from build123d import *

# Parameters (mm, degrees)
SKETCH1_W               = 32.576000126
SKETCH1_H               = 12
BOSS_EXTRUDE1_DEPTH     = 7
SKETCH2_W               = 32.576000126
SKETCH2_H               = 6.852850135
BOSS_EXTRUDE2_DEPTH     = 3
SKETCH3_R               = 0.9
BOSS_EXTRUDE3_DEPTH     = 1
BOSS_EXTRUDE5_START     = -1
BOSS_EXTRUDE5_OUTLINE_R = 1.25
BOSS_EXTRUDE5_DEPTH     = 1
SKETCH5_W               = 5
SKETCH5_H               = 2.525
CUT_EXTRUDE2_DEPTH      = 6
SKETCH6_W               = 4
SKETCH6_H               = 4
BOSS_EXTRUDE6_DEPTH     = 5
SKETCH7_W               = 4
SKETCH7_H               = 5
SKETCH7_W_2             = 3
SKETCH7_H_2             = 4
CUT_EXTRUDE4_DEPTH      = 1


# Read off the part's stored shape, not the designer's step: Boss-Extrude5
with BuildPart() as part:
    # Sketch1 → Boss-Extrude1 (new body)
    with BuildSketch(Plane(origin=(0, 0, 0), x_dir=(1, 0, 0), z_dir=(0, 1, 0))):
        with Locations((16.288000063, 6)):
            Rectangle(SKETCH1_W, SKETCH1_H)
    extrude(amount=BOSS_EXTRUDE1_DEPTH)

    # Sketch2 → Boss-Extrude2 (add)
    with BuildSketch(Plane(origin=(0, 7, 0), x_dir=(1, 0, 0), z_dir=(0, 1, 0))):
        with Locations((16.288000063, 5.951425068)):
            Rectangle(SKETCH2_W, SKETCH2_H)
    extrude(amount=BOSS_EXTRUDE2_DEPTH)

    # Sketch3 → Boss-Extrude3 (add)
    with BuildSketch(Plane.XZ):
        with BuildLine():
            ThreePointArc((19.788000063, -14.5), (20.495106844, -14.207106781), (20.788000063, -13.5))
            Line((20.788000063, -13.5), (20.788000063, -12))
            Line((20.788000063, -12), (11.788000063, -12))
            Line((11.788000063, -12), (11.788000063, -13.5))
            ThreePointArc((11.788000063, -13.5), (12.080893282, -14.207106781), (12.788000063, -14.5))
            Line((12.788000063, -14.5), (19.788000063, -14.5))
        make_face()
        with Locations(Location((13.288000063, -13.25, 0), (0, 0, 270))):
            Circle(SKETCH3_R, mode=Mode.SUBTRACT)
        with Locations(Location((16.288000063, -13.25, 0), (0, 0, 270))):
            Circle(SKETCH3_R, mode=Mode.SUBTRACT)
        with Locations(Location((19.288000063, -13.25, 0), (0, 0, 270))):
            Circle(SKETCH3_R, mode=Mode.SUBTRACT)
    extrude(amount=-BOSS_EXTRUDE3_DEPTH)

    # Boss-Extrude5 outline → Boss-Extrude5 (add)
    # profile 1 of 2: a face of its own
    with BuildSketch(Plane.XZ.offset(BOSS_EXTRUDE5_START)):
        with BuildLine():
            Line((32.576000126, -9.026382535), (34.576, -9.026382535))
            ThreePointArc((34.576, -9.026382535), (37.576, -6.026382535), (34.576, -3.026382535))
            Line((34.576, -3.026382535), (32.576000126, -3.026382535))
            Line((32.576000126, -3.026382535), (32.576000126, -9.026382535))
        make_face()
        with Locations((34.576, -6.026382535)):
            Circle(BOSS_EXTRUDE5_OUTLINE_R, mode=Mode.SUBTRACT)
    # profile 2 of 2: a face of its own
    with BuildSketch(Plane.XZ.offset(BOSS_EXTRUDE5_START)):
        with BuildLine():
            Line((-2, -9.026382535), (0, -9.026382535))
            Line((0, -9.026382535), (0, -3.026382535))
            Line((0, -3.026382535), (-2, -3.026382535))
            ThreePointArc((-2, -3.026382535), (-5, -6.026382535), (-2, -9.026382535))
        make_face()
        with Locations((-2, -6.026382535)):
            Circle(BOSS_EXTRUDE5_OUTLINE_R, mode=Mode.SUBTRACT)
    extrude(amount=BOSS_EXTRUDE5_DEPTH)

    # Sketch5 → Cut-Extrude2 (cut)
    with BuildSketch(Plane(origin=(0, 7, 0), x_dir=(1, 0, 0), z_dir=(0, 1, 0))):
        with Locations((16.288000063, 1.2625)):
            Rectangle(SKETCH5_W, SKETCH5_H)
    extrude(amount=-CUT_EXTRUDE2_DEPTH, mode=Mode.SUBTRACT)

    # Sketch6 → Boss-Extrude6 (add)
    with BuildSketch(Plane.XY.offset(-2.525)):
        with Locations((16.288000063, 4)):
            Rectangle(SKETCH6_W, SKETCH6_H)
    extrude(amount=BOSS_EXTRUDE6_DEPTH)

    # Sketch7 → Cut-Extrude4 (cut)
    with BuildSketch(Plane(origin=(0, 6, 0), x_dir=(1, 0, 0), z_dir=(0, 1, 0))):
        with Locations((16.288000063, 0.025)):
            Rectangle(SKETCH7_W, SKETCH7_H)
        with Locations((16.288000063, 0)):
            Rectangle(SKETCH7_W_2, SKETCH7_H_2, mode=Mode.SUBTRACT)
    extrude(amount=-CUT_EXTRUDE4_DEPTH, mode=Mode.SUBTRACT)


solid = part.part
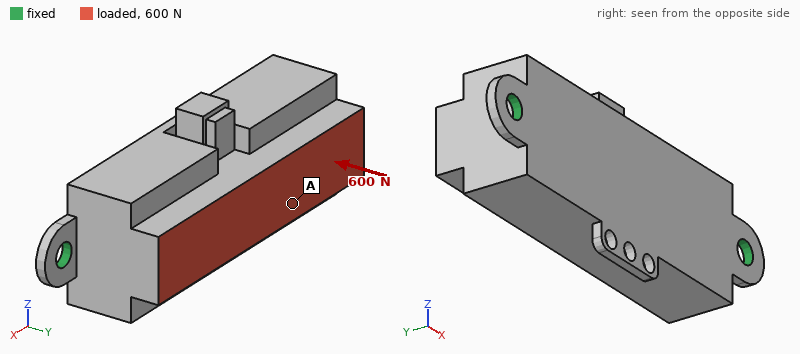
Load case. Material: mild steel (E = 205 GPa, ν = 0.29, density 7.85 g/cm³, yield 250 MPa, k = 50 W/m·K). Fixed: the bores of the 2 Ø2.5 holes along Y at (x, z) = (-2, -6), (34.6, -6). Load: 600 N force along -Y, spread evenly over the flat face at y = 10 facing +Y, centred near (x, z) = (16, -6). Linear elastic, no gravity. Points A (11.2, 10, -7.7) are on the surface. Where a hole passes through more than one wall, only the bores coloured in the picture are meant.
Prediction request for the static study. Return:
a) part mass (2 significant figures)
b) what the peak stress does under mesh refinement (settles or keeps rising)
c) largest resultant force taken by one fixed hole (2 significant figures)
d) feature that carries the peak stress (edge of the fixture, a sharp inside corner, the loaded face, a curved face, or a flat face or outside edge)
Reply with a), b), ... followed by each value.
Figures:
a) 27 g
b) keeps rising
c) 370 N
d) edge of the fixture
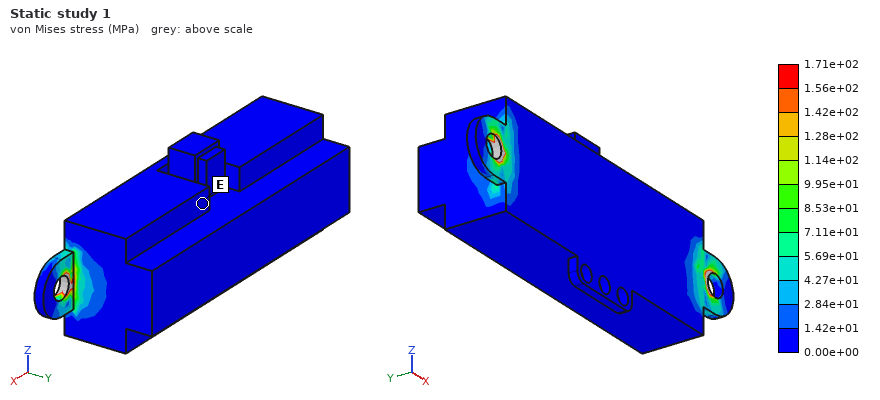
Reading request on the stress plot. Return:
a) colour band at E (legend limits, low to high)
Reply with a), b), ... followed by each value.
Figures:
a) 0.00e+00 to 1.42e+01 MPa
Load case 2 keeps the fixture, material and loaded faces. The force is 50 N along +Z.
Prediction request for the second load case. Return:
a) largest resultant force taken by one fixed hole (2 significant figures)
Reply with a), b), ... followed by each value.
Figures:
a) 25 N
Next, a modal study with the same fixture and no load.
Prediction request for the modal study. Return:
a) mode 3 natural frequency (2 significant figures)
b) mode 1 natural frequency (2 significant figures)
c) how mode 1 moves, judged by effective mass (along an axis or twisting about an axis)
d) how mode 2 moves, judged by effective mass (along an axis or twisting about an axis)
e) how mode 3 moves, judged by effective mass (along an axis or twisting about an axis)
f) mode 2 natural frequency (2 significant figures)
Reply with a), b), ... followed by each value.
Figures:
a) 18 kHz
b) 3400 Hz
c) along Z
d) along Y
e) along Z
f) 12 kHz
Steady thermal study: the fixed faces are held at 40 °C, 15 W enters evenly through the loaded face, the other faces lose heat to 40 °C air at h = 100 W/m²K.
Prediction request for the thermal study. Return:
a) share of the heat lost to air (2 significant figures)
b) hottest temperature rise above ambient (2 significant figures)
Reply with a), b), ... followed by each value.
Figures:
a) 42 %
b) 48 K
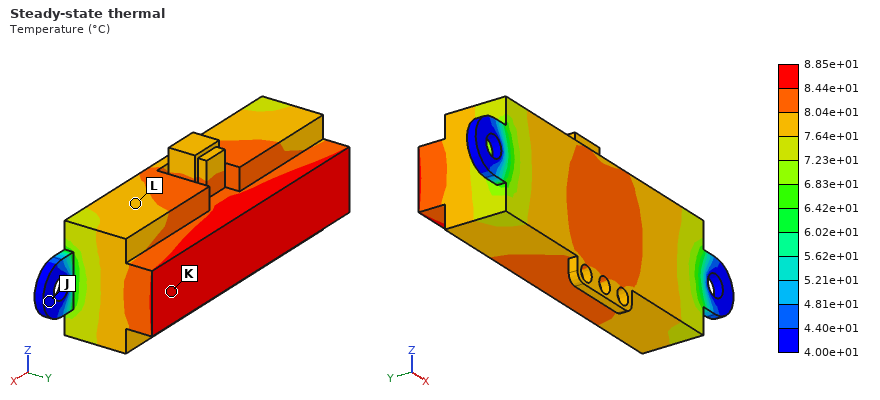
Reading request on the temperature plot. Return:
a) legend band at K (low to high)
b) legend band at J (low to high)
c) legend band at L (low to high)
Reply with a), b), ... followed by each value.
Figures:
a) 8.44e+01 to 8.85e+01 °C
b) 4.00e+01 to 4.40e+01 °C
c) 7.64e+01 to 8.04e+01 °C
